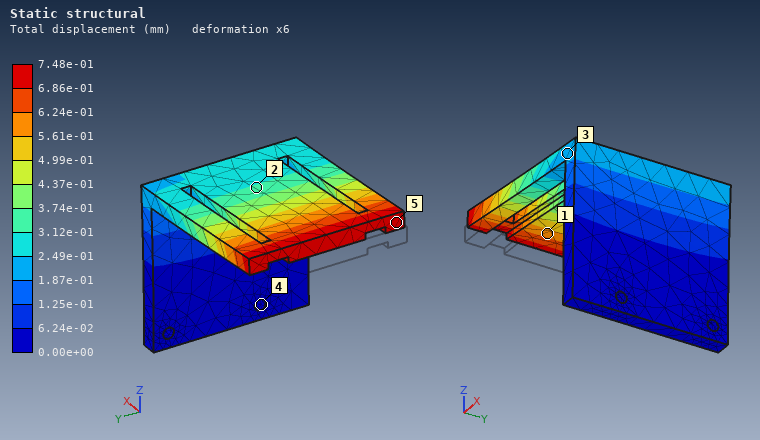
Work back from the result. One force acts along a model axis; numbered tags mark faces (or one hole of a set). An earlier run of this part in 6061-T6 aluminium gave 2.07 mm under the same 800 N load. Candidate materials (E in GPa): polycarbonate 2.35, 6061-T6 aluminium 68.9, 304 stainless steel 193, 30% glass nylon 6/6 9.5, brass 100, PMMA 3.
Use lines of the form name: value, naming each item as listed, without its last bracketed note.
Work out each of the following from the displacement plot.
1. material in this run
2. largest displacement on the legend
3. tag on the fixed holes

material in this run: 304 stainless steel
largest displacement on the legend: 7.48e-01 mm
tag on the fixed holes: 4
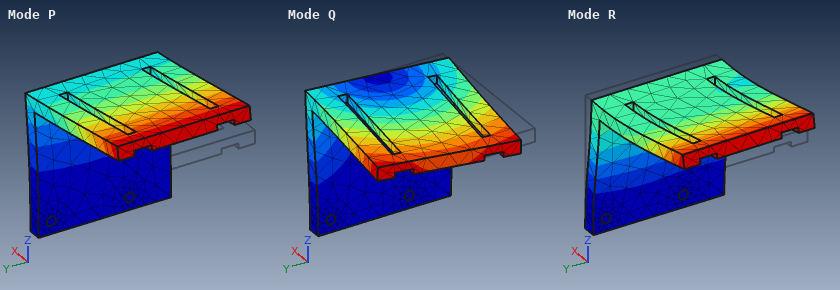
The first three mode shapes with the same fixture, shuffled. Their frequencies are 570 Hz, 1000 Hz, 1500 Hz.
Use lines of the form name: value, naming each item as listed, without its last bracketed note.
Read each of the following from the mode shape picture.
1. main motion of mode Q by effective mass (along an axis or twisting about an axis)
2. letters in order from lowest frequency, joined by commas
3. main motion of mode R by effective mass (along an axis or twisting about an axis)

main motion of mode Q by effective mass: along Y
letters in order from lowest frequency, joined by commas: P, Q, R
main motion of mode R by effective mass: along X
